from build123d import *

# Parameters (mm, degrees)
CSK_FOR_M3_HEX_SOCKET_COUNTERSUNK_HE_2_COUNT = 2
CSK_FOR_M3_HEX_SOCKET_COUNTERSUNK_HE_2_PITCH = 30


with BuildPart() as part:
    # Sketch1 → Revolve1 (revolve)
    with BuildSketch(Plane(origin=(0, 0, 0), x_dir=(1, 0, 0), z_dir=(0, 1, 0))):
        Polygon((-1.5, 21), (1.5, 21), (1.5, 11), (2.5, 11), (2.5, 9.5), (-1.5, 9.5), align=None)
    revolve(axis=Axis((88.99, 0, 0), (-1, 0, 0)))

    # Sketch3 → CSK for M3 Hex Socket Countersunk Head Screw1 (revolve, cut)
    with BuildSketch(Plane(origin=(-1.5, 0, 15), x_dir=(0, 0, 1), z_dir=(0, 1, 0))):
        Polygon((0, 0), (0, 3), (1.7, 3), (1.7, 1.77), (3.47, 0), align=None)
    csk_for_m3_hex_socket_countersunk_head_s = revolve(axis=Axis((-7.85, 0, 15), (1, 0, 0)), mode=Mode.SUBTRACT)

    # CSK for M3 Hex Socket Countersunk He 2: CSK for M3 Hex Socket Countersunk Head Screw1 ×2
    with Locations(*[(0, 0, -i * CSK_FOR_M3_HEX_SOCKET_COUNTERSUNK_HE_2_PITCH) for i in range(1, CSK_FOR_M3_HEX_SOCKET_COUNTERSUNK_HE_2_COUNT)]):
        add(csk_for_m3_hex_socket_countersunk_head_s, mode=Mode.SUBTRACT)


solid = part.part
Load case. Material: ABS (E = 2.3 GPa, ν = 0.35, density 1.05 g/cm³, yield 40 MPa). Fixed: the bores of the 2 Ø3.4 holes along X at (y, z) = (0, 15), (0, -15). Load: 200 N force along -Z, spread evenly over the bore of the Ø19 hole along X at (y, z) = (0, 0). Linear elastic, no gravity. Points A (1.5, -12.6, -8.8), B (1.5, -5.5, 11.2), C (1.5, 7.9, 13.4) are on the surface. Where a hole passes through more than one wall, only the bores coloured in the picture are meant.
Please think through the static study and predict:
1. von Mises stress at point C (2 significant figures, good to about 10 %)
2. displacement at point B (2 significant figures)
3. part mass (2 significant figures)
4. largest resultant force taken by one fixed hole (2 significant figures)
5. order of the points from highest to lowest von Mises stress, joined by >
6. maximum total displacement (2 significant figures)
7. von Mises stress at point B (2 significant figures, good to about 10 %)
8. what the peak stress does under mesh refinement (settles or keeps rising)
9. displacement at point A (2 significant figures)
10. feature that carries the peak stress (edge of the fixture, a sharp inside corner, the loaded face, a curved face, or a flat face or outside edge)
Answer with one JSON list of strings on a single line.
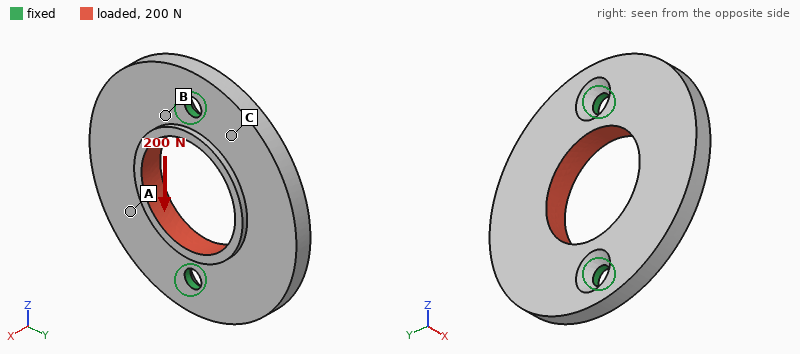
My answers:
["2.1 MPa", "15 µm", "3.5 g", "100 N", "B > C > A", "28 µm", "3.6 MPa", "keeps rising", "23 µm", "edge of the fixture"]
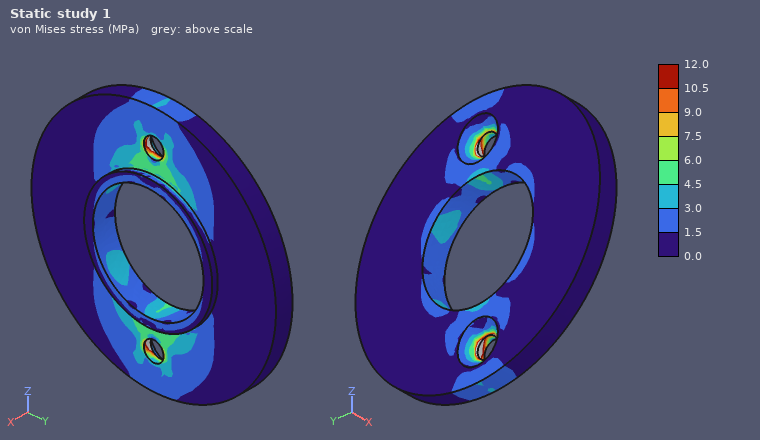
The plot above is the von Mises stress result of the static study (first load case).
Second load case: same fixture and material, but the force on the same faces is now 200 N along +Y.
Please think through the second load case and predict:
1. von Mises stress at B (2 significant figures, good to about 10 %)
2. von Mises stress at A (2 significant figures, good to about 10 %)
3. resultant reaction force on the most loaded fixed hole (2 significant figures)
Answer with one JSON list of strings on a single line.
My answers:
["2.7 MPa", "1.4 MPa", "100 N"]
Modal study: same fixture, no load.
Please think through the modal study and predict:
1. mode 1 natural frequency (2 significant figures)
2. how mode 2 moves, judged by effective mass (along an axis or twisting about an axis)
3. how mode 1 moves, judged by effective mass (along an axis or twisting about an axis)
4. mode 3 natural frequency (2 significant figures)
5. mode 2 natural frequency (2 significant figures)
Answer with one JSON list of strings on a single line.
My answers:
["1100 Hz", "along X", "twisting about Z", "3100 Hz", "1500 Hz"]
